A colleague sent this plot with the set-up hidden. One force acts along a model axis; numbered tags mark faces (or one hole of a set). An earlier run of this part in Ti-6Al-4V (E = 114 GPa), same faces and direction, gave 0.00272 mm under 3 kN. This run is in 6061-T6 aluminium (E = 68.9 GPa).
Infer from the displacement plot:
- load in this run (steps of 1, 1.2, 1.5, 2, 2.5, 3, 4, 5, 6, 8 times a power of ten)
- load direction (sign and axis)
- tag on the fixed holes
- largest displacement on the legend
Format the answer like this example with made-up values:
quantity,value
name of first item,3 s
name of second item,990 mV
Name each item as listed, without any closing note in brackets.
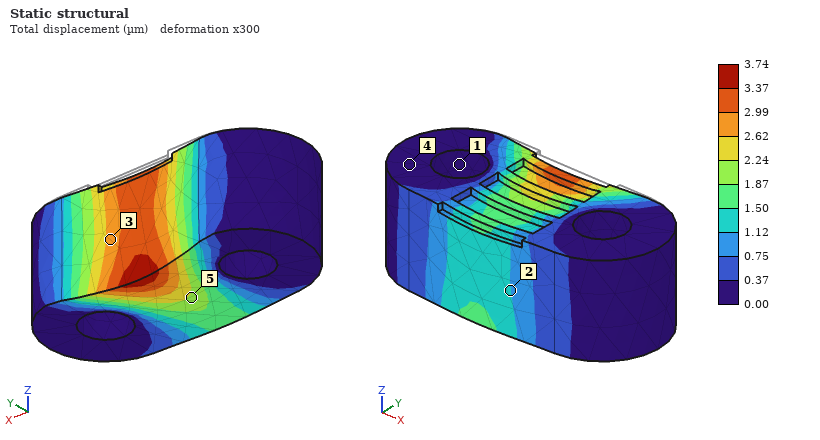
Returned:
quantity,value
load in this run,2.5 kN
load direction,-Y
tag on the fixed holes,1
largest displacement on the legend,3.74 µm
